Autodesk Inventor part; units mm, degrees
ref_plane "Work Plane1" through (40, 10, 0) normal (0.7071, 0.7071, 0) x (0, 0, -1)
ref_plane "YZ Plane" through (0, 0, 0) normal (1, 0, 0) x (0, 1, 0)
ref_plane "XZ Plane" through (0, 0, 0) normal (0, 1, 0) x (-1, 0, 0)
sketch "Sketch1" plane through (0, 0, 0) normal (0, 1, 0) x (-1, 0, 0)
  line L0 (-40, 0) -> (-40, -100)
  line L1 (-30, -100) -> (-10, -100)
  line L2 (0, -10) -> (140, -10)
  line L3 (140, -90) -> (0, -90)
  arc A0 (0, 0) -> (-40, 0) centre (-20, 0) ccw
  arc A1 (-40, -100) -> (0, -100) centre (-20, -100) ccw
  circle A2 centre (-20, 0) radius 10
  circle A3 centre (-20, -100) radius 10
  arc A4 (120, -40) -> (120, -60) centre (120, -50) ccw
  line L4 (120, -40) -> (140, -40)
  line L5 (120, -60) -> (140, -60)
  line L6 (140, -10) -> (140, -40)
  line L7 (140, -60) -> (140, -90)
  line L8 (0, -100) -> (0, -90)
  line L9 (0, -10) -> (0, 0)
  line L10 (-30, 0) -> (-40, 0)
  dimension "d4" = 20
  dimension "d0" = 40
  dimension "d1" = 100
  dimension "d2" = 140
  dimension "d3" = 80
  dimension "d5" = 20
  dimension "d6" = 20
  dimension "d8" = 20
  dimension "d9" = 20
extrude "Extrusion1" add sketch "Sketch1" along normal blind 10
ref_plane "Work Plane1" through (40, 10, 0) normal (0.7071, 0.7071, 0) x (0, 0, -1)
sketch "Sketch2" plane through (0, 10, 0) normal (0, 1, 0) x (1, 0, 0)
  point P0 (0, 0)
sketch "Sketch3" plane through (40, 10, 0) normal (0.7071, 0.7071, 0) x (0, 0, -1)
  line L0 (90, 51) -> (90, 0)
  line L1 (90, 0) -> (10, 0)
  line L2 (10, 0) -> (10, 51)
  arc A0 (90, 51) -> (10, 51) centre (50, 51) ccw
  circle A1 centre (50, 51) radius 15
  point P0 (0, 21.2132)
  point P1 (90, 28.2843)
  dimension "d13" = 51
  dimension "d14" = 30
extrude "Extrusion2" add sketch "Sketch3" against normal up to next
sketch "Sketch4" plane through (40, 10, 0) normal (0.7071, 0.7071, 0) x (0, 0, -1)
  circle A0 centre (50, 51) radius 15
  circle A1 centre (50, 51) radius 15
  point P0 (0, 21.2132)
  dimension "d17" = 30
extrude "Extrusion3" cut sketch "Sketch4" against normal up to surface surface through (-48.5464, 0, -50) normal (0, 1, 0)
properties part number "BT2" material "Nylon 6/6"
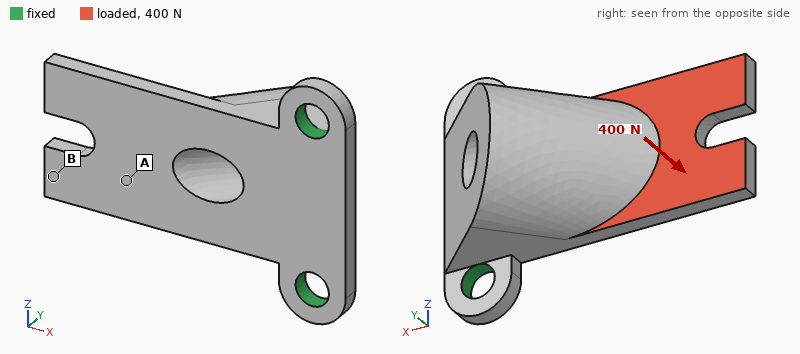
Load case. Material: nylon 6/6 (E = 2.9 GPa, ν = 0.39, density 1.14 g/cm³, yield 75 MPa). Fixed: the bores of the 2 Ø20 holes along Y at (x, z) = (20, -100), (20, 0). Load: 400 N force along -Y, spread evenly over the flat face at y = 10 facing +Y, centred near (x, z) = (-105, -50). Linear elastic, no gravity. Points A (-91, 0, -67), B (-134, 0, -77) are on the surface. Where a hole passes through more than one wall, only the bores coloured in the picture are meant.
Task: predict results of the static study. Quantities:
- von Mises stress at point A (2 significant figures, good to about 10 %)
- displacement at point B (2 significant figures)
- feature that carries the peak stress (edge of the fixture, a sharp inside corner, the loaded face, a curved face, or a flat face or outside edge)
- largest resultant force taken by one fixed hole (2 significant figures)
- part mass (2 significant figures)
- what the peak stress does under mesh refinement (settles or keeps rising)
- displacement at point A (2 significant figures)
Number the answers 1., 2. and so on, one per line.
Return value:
1. 4.4 MPa
2. 2.2 mm
3. edge of the fixture
4. 300 N
5. 430 g
6. keeps rising
7. 1.3 mm
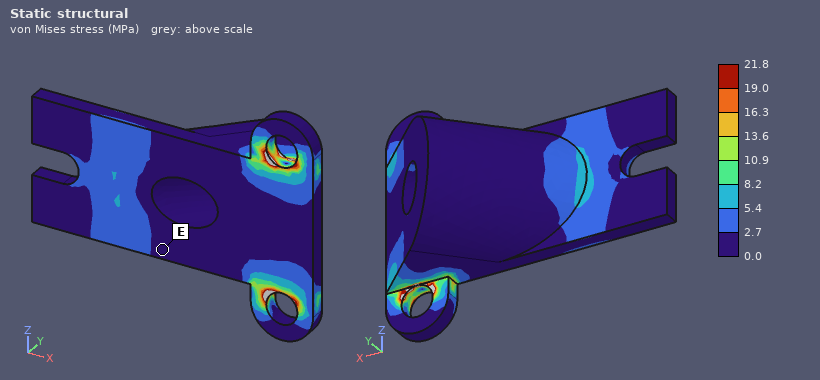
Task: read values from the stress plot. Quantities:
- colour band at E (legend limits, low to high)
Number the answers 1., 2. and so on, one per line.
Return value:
1. 0.0 to 2.7 MPa
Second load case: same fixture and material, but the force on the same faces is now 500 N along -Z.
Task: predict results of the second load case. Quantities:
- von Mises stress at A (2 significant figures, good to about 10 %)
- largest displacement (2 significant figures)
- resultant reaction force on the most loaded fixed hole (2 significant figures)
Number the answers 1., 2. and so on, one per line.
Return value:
1. 0.65 MPa
2. 0.29 mm
3. 730 N
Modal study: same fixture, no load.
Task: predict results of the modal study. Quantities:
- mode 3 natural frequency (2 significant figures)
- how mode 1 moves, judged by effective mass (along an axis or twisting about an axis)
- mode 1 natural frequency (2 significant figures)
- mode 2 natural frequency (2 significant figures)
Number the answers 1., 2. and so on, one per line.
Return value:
1. 850 Hz
2. along Y
3. 250 Hz
4. 790 Hz
